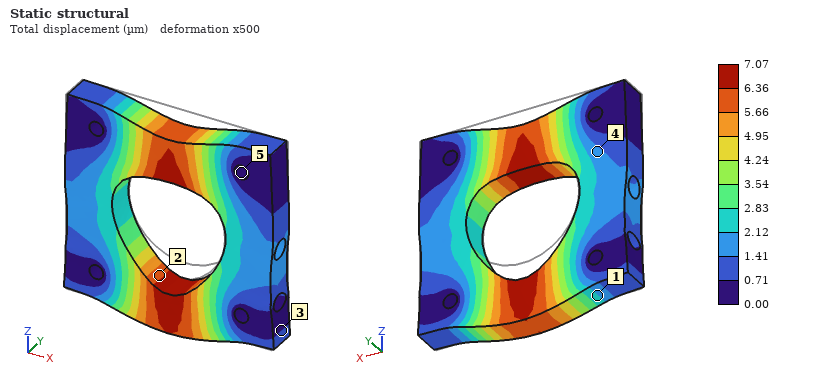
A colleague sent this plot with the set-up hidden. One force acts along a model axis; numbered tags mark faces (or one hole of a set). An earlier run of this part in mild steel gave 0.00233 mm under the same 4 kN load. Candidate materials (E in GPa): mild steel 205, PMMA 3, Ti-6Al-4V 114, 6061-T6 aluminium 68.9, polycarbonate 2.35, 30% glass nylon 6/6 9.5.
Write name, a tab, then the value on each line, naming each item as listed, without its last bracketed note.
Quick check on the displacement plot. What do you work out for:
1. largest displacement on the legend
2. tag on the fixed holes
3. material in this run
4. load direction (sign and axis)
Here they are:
largest displacement on the legend	7.07 µm
tag on the fixed holes	5
material in this run	6061-T6 aluminium
load direction	-Z
